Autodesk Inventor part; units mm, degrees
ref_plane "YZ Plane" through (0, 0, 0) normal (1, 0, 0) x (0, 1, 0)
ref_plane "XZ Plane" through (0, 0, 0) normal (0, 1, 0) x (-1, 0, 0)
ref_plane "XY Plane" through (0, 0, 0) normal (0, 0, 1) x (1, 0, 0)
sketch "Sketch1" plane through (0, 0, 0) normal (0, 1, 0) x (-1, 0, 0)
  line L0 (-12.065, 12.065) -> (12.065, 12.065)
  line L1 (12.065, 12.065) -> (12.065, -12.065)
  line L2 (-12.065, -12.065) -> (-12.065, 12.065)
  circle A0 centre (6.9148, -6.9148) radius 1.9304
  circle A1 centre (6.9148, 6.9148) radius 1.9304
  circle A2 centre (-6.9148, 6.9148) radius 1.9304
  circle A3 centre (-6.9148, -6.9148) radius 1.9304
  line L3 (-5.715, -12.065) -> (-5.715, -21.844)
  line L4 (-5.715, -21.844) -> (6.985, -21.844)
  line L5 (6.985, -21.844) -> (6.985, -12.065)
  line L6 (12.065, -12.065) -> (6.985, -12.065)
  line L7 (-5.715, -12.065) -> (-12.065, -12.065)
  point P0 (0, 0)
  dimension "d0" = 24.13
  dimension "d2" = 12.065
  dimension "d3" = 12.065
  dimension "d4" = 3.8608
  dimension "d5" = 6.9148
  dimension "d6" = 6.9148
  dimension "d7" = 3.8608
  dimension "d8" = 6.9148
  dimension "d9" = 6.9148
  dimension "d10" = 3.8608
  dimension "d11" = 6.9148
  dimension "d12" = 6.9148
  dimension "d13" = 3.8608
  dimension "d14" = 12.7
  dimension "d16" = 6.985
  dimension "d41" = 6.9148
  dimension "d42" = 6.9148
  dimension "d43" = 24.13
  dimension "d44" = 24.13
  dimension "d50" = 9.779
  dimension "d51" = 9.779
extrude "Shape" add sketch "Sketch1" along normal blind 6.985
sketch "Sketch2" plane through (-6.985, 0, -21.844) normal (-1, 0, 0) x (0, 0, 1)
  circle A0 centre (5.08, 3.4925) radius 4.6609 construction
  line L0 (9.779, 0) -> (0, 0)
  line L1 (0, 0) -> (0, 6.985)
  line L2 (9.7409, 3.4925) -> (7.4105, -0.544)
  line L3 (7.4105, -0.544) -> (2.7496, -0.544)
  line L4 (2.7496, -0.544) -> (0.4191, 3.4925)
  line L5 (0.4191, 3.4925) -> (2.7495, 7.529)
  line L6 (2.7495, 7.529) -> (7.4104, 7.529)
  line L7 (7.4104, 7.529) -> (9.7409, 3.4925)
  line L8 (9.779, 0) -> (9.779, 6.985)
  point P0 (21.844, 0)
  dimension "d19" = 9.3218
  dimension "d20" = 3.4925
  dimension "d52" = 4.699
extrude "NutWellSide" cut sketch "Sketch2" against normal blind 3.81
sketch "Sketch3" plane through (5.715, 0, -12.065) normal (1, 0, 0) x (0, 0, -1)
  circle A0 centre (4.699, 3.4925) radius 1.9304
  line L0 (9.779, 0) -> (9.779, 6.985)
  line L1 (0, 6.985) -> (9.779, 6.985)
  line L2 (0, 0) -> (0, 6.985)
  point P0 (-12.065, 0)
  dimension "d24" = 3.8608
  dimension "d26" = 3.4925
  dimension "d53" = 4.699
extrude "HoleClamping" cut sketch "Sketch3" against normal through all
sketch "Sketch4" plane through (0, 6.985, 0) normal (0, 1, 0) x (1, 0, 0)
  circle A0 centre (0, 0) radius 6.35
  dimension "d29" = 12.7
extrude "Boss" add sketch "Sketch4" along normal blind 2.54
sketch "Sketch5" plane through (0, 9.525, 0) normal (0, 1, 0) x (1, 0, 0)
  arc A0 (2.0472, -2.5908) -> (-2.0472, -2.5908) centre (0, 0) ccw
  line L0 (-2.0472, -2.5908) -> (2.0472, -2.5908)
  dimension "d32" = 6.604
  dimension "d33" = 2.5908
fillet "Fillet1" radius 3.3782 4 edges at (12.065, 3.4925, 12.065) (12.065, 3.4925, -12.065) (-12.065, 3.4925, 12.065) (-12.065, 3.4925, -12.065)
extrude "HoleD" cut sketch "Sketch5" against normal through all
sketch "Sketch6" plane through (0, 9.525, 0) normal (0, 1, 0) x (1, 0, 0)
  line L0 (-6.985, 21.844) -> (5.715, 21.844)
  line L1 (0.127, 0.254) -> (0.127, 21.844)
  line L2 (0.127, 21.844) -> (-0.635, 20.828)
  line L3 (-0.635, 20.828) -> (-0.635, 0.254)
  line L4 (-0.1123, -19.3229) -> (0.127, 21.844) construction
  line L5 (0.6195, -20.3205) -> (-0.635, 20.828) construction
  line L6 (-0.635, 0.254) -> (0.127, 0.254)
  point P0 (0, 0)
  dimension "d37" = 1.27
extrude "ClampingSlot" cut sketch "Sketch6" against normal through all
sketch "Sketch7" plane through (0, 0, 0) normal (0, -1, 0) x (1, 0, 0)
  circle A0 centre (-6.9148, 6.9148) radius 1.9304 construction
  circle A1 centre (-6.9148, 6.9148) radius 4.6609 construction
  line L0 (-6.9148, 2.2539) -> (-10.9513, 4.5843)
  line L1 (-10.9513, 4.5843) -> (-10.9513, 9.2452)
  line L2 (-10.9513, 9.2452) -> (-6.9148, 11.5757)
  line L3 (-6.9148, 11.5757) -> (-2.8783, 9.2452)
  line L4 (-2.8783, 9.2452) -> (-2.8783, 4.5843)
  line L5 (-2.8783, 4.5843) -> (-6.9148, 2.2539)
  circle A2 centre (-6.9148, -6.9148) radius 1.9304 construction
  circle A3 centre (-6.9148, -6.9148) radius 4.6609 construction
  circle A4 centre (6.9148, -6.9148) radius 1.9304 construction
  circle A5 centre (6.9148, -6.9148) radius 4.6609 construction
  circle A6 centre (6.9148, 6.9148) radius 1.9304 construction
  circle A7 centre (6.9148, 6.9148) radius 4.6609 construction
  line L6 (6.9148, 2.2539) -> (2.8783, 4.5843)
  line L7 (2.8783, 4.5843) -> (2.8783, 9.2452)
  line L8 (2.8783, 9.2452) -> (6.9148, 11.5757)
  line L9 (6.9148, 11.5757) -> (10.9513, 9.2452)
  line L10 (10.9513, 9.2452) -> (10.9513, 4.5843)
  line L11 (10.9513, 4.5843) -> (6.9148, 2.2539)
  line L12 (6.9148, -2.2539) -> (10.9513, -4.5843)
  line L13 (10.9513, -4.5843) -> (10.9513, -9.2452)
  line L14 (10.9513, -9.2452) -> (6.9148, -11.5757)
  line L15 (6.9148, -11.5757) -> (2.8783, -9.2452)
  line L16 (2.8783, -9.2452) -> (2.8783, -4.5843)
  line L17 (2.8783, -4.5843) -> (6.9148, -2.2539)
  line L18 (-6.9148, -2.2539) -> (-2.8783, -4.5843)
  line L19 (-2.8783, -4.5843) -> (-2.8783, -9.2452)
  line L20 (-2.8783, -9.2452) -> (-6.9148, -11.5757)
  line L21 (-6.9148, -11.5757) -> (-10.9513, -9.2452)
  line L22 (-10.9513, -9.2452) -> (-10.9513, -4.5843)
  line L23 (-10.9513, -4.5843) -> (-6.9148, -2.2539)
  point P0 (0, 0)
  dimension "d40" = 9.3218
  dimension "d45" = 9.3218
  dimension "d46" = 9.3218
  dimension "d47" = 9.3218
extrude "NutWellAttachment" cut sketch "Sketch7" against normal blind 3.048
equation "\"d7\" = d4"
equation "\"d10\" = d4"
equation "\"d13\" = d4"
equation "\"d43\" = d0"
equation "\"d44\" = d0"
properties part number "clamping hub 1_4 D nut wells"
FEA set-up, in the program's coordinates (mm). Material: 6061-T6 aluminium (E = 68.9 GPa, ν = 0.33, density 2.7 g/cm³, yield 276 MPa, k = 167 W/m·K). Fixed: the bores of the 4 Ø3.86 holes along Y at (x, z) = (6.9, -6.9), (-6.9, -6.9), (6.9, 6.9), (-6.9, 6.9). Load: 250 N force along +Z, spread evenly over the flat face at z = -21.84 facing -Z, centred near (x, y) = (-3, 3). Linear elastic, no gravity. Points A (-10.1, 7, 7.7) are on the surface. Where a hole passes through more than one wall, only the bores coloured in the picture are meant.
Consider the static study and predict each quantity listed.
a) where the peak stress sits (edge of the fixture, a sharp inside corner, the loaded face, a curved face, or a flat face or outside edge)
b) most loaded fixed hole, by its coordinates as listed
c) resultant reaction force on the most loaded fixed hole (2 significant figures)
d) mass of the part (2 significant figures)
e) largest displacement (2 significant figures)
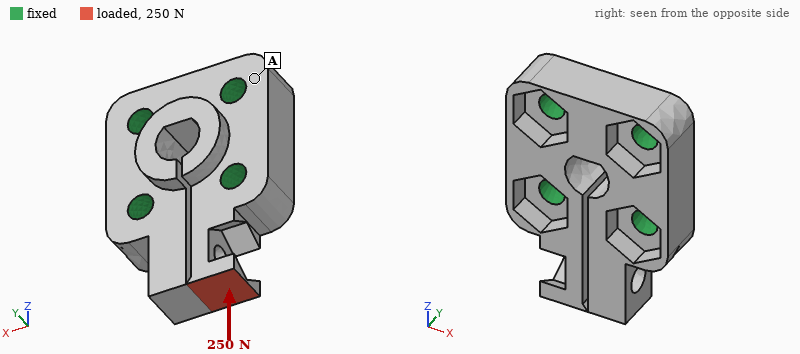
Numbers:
a curved face
(-6.9, -6.9)
240 N
9.8 g
33 µm
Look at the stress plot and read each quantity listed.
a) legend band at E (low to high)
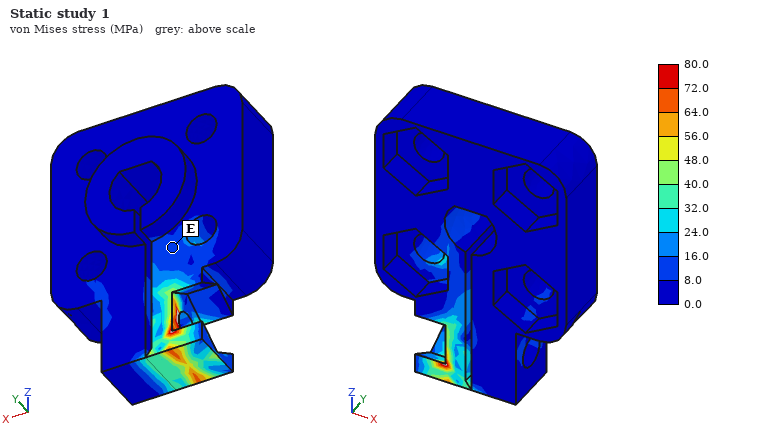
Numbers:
8.0 to 16.0 MPa
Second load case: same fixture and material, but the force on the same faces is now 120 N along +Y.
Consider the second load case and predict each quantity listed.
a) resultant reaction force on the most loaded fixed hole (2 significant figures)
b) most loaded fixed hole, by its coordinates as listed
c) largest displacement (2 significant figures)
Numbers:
100 N
(-6.9, -6.9)
33 µm
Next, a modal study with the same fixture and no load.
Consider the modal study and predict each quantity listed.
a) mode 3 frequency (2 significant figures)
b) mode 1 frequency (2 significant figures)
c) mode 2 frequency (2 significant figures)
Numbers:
29 kHz
17 kHz
23 kHz
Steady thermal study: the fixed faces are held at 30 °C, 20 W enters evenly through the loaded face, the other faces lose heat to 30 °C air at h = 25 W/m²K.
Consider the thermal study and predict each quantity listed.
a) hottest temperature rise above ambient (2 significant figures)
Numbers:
81 K
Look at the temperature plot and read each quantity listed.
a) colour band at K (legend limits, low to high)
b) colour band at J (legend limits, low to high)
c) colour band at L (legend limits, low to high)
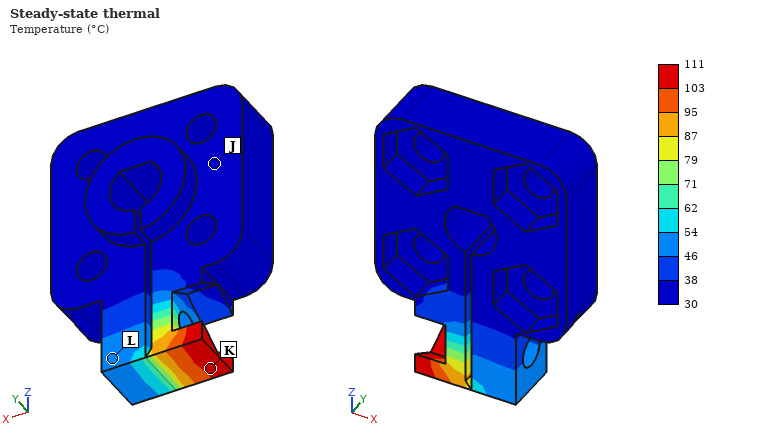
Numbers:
103 to 111 °C
30 to 38 °C
46 to 54 °C
